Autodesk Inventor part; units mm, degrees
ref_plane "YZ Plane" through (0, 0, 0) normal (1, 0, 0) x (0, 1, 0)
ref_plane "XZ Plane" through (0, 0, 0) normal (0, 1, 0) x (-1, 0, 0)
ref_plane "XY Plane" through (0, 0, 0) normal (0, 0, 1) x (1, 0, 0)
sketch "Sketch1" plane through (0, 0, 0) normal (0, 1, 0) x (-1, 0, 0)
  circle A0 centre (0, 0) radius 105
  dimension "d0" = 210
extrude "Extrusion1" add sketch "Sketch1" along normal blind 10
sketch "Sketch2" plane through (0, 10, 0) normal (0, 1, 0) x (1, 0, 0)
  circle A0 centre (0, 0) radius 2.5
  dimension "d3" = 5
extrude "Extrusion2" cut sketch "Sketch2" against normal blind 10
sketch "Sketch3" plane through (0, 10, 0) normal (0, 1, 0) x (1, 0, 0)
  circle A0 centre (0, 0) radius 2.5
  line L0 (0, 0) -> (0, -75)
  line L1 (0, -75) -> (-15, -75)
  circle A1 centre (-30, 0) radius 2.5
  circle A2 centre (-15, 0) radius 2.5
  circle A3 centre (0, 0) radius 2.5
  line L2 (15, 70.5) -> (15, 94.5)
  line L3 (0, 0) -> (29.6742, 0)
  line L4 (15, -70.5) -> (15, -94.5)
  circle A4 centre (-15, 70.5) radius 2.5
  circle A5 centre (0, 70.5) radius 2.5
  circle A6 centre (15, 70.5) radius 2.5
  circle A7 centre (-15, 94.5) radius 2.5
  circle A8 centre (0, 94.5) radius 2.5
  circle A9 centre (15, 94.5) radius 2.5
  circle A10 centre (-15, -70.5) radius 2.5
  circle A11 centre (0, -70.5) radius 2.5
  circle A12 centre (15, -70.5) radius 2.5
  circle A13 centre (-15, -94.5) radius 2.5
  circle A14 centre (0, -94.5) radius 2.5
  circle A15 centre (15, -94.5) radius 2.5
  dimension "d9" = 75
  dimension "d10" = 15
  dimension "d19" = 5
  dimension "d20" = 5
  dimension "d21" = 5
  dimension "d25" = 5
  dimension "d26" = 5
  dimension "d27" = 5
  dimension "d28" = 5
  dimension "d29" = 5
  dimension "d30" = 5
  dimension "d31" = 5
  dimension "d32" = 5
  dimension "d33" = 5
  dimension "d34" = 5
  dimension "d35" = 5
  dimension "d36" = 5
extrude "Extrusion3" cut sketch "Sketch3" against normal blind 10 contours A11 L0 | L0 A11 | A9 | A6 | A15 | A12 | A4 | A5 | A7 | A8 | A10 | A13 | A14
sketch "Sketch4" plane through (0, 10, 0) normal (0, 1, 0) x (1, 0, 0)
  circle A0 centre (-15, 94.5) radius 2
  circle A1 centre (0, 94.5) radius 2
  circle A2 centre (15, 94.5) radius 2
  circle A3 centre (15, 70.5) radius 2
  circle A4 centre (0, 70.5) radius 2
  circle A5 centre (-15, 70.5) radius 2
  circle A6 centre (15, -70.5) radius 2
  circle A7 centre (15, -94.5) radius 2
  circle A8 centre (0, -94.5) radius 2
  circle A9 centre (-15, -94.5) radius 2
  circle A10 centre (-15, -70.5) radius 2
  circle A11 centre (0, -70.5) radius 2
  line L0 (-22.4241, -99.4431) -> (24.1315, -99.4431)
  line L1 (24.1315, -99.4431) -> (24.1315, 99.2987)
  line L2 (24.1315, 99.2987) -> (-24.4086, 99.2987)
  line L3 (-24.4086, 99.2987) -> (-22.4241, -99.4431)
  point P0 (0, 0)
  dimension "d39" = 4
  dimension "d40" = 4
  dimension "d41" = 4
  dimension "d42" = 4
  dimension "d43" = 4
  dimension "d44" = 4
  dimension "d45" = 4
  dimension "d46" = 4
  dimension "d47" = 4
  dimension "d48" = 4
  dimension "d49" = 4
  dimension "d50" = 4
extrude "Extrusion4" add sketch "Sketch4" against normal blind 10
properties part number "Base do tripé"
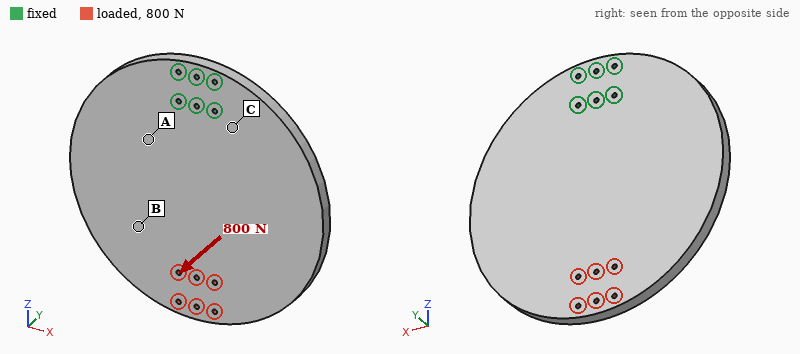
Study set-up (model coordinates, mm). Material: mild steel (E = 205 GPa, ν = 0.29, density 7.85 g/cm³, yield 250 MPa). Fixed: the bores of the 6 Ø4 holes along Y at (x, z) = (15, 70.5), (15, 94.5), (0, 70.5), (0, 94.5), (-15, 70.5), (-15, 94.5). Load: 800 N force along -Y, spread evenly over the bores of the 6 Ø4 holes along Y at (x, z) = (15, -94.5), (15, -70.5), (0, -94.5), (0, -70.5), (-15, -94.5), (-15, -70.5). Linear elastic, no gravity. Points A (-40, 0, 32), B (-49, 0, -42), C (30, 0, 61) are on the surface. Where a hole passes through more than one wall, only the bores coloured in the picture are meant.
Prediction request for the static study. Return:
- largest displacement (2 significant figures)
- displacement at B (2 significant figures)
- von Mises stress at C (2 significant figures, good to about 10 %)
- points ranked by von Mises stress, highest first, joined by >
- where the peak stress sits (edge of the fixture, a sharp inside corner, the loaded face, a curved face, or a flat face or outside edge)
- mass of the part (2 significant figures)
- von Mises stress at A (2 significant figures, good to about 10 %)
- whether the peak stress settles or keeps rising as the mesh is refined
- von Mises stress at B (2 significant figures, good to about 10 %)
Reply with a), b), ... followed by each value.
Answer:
a) 0.48 mm
b) 0.25 mm
c) 43 MPa
d) C > A > B
e) edge of the fixture
f) 2.7 kg
g) 29 MPa
h) keeps rising
i) 12 MPa
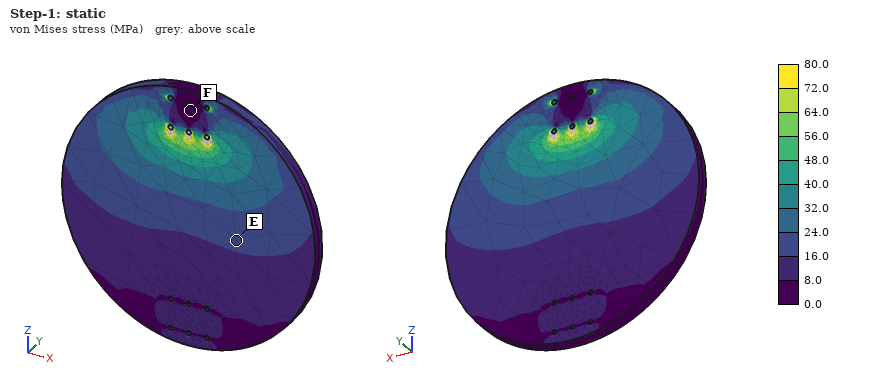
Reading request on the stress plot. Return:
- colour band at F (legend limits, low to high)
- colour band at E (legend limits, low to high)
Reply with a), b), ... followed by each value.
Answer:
a) 0.0 to 8.0 MPa
b) 16.0 to 24.0 MPa
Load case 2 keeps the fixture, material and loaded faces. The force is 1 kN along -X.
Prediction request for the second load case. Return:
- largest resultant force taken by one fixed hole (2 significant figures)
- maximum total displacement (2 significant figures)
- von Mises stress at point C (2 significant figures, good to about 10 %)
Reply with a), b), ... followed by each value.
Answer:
a) 2.3 kN
b) 15 µm
c) 4.6 MPa
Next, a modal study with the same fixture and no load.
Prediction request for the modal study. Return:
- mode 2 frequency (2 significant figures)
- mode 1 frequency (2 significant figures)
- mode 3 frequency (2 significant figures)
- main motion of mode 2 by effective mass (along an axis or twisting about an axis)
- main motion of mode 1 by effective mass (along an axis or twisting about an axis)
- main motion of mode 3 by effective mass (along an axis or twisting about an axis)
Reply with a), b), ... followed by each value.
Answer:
a) 490 Hz
b) 270 Hz
c) 1100 Hz
d) twisting about Z
e) along Y
f) along Y
